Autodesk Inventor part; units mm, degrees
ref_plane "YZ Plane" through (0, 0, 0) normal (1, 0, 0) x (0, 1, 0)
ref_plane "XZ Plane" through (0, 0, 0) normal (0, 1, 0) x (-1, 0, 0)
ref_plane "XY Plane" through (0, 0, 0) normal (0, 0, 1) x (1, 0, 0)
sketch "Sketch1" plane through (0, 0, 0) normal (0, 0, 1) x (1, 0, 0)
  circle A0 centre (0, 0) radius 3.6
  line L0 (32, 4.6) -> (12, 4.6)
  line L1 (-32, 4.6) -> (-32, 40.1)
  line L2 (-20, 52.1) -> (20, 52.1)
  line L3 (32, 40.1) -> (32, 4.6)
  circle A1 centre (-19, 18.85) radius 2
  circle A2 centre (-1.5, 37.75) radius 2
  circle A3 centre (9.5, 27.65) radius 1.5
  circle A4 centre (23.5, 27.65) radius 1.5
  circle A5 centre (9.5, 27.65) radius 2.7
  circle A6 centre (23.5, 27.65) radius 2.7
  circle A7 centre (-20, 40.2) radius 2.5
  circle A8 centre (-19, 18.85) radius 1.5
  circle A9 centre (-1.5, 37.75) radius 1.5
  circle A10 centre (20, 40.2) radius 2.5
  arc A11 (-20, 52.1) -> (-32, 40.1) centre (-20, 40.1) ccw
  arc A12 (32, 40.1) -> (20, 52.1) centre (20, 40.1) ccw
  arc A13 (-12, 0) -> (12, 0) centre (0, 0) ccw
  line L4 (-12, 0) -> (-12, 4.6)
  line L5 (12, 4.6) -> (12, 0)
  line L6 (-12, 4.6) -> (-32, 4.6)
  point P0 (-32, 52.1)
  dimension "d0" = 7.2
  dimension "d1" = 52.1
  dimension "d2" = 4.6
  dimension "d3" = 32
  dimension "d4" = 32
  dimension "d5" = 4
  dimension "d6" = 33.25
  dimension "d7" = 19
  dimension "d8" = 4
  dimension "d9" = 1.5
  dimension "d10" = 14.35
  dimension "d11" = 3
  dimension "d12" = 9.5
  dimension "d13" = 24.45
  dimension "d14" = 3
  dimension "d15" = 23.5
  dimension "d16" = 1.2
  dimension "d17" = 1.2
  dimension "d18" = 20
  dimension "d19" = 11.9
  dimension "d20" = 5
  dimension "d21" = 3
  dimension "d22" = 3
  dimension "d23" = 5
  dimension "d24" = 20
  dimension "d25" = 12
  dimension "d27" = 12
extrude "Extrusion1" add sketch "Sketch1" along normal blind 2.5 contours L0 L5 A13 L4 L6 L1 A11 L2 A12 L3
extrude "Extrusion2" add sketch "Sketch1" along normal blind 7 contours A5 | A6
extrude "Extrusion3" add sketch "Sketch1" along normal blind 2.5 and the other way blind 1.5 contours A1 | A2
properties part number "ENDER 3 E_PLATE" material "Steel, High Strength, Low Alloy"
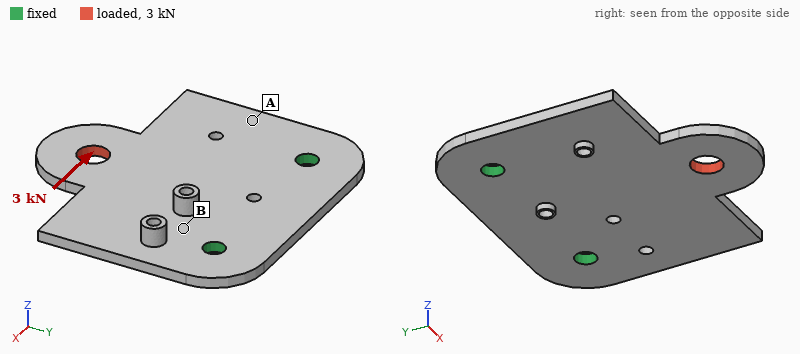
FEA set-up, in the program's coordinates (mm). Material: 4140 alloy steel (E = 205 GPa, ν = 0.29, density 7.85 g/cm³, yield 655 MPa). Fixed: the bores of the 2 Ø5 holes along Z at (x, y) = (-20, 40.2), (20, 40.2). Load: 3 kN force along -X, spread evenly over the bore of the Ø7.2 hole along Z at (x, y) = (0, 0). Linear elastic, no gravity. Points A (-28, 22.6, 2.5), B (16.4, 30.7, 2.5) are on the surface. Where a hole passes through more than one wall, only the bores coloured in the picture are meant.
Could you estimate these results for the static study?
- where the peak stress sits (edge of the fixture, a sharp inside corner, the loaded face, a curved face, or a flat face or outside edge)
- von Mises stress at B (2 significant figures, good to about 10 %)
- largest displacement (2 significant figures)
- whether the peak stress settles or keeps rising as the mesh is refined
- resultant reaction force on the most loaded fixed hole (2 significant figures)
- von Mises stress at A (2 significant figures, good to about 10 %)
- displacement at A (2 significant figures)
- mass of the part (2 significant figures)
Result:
edge of the fixture
68 MPa
34 µm
keeps rising
3.2 kN
29 MPa
11 µm
64 g
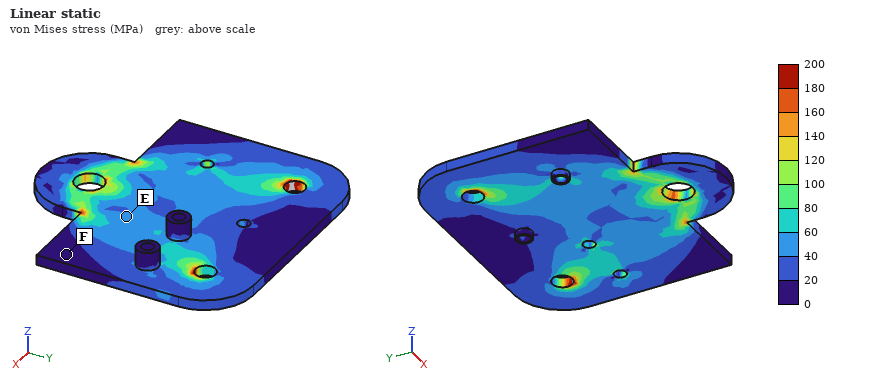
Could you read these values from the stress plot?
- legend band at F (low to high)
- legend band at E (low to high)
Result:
0 to 20 MPa
40 to 60 MPa
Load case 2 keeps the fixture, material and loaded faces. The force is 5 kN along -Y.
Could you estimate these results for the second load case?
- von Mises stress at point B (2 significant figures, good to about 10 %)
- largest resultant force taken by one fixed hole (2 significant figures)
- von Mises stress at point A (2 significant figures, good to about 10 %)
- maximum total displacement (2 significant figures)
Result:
62 MPa
2.6 kN
14 MPa
18 µm
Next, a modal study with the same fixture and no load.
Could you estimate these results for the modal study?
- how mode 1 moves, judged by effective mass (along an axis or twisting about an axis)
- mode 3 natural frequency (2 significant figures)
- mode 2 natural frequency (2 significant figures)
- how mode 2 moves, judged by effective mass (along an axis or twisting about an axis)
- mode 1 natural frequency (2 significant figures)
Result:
along Z
4100 Hz
2700 Hz
twisting about Y
1100 Hz
